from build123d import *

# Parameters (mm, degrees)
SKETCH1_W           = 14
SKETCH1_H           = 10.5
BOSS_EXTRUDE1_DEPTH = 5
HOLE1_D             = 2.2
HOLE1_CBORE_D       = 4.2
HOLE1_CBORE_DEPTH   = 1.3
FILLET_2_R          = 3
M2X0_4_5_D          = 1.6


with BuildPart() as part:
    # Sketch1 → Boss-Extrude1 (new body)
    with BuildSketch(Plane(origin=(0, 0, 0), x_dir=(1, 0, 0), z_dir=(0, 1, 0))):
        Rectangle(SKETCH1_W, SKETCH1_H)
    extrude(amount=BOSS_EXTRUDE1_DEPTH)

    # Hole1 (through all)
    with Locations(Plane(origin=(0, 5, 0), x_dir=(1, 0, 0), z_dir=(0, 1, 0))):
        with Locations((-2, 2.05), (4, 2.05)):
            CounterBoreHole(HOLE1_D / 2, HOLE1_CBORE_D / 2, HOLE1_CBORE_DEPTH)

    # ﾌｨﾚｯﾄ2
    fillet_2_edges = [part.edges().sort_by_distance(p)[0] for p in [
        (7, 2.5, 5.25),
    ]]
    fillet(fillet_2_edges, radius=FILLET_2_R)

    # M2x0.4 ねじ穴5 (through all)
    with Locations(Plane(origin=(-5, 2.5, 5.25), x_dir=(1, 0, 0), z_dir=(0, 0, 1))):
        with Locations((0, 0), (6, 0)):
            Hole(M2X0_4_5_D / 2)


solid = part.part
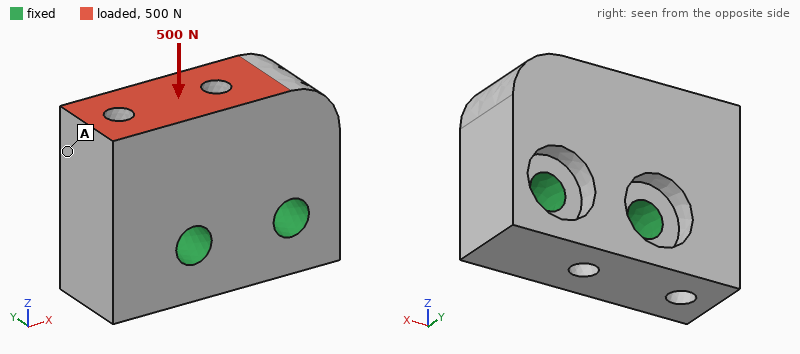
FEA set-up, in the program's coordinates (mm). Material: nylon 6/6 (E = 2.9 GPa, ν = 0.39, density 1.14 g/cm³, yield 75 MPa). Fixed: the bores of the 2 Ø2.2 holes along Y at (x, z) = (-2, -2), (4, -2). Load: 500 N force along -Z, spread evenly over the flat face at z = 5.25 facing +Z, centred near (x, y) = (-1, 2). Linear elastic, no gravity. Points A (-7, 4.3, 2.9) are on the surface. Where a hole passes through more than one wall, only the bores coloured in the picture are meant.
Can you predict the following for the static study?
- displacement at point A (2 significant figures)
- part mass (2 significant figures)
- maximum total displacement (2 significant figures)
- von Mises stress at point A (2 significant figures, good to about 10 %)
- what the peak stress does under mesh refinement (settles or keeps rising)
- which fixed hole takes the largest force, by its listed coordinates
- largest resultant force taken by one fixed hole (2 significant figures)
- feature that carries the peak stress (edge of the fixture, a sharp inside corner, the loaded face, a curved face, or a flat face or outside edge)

66 µm
0.71 g
82 µm
9.4 MPa
keeps rising
(-2, -2)
410 N
edge of the fixture
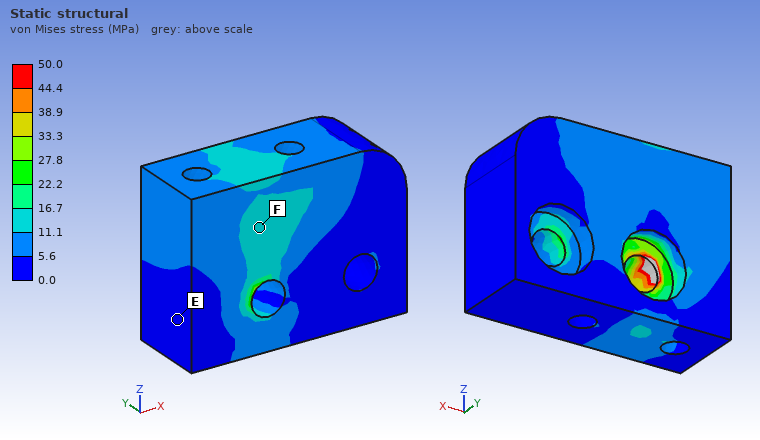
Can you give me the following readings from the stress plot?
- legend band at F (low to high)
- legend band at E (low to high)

11.1 to 16.7 MPa
0.0 to 5.6 MPa
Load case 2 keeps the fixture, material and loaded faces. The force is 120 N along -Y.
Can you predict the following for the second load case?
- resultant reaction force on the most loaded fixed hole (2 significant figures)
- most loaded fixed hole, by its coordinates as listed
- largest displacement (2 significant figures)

89 N
(-2, -2)
0.12 mm
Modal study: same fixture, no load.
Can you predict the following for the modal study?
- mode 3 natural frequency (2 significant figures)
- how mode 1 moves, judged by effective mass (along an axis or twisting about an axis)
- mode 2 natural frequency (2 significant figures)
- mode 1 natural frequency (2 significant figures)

20 kHz
along Y
20 kHz
15 kHz
